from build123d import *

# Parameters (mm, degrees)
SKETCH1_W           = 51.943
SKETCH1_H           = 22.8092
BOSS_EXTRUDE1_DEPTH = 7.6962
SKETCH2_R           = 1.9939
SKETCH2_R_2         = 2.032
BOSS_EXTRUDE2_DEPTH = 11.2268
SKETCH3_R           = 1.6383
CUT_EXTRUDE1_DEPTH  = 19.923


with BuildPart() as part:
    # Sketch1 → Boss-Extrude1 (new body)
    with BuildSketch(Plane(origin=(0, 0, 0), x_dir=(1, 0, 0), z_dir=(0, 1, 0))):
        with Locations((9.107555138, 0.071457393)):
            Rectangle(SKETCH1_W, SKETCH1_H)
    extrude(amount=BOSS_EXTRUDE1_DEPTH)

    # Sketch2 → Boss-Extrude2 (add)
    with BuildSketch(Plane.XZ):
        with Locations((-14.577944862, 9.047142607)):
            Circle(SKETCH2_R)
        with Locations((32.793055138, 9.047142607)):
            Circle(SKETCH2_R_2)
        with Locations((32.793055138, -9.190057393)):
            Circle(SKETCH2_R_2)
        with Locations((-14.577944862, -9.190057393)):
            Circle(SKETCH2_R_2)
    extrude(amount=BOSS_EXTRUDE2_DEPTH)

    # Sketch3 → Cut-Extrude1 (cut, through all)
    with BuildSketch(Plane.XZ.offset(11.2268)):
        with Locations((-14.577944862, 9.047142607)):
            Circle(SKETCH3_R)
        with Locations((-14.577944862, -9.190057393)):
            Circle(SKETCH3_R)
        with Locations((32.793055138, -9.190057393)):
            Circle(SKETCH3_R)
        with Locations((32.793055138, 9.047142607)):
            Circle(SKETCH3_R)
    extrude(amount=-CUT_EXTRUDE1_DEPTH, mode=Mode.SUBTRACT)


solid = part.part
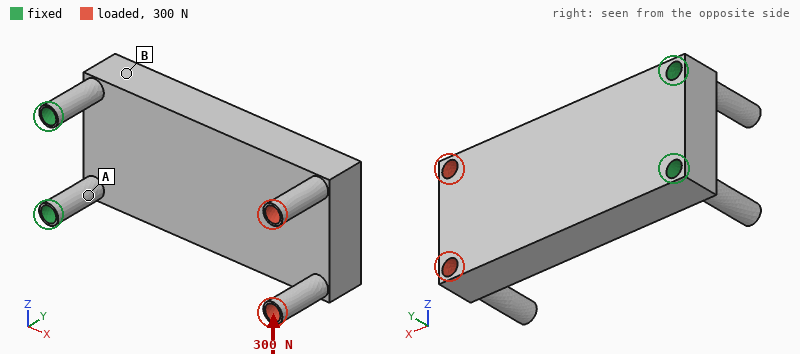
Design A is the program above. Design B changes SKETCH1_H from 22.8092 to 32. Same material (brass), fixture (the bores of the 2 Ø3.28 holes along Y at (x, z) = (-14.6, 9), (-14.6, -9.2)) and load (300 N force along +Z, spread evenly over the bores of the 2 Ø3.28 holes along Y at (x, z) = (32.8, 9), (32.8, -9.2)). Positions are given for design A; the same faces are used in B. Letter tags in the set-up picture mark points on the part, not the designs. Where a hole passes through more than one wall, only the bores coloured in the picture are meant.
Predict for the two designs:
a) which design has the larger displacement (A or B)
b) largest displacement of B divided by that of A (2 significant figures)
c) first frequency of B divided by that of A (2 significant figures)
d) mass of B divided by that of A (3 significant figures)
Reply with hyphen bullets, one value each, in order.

- A
- 0.77
- 0.99
- 1.41
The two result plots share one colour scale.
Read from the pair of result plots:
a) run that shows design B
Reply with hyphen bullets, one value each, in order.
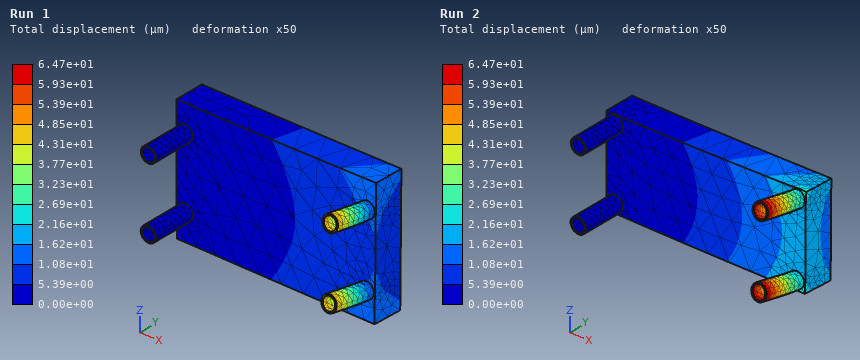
- Run 1
